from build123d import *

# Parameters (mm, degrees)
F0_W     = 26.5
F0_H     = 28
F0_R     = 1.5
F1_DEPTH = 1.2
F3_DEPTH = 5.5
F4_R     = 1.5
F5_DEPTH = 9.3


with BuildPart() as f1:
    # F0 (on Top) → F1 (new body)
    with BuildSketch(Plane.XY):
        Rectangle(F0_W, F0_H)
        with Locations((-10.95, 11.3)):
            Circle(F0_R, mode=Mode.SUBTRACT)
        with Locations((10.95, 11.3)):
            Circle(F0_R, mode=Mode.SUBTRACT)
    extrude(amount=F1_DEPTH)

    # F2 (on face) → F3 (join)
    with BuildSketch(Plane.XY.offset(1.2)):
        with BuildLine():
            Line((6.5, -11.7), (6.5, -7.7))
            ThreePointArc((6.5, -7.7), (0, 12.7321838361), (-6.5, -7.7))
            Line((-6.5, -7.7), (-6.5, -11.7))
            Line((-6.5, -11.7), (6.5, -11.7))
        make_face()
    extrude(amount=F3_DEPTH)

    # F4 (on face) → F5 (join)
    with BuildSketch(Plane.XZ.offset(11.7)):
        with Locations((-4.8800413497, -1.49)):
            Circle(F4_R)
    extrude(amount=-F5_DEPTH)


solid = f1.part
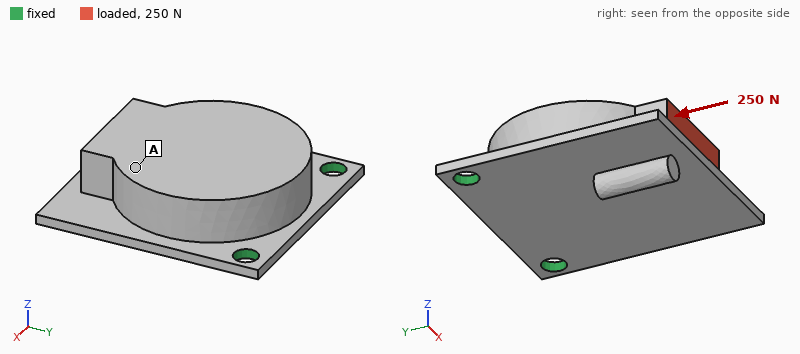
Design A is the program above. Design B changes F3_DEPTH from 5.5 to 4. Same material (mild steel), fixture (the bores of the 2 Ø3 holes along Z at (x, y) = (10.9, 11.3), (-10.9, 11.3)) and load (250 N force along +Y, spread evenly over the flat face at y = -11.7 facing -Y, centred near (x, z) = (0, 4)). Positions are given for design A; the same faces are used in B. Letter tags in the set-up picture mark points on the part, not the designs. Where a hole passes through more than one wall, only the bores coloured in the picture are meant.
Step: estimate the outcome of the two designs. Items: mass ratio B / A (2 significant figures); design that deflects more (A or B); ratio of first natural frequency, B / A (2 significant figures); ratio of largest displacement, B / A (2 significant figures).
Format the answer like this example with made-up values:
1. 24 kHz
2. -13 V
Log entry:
1. 0.80
2. A
3. 1.1
4. 0.80
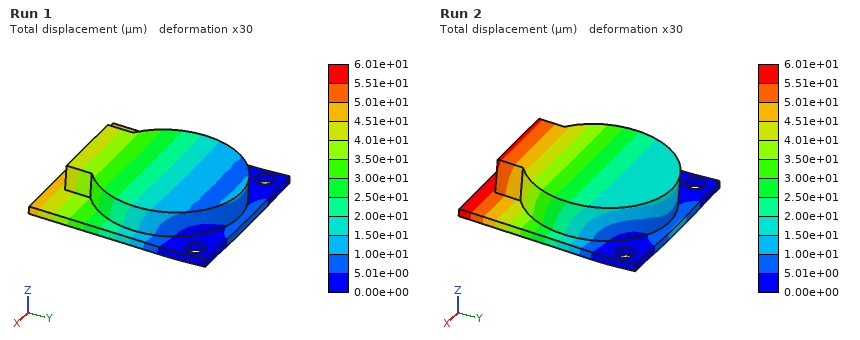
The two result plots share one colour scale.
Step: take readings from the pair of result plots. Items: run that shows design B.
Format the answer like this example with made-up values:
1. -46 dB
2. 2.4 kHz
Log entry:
1. Run 1
